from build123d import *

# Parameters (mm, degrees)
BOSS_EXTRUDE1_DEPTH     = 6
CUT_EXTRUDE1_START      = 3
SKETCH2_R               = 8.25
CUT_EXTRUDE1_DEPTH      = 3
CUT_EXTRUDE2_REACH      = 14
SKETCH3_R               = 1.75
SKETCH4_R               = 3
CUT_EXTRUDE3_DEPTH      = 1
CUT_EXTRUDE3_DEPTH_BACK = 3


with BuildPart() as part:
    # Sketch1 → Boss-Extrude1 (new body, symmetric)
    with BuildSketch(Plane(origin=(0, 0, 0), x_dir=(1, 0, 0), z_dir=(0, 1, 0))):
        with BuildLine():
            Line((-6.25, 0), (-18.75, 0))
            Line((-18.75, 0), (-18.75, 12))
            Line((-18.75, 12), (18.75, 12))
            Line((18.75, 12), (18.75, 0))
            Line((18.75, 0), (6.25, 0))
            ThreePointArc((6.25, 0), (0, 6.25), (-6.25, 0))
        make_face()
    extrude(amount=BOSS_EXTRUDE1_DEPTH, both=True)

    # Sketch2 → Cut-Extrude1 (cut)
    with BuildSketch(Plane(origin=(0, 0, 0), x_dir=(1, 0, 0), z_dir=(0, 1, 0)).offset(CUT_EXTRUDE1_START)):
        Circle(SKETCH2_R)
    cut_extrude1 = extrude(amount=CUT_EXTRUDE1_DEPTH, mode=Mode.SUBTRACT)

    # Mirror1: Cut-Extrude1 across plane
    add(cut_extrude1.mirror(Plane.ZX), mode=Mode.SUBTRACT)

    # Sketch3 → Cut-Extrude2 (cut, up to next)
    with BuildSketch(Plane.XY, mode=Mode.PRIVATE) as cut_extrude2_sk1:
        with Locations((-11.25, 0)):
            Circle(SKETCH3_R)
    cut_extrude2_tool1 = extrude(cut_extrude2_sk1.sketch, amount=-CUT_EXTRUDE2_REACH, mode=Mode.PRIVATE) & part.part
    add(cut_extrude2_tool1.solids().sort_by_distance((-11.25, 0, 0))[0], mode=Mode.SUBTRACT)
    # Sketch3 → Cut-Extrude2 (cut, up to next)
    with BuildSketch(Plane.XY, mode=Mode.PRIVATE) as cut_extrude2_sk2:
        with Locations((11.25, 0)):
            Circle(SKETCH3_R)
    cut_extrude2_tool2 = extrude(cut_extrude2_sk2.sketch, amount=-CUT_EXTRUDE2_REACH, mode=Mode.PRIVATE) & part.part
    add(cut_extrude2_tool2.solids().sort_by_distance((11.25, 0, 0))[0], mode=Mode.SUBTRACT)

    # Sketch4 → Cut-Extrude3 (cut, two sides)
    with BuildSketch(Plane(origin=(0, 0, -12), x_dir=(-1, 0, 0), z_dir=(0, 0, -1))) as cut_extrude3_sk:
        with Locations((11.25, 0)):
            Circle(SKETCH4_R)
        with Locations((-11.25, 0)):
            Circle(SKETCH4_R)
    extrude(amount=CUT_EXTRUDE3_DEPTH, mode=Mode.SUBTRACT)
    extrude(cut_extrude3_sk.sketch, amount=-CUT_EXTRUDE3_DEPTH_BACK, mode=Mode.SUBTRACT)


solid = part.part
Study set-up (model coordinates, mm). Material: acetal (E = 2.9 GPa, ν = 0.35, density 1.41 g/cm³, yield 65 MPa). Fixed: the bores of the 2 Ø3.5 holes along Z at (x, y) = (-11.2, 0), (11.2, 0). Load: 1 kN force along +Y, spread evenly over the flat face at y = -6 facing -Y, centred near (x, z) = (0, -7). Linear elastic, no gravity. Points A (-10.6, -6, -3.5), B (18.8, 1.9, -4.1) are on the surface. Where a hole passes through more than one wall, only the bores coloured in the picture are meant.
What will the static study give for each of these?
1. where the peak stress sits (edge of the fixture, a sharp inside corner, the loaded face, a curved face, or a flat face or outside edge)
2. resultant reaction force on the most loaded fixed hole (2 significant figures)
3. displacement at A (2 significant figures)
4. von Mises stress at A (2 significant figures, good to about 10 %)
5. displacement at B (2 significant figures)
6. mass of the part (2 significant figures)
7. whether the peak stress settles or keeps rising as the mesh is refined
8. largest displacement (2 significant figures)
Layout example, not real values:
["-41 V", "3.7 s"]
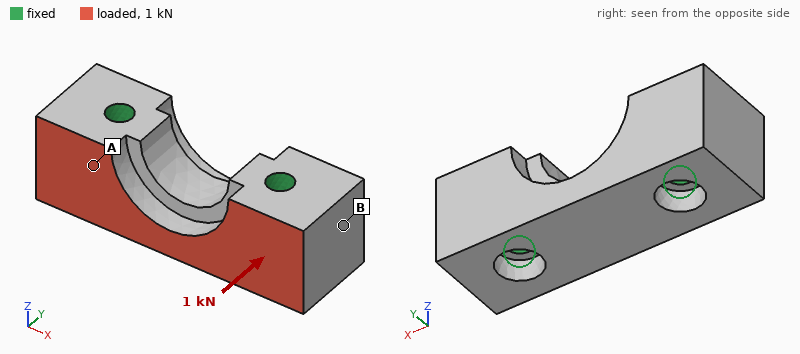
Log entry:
["edge of the fixture", "500 N", "8.7 µm", "5.6 MPa", "12 µm", "5.7 g", "keeps rising", "38 µm"]
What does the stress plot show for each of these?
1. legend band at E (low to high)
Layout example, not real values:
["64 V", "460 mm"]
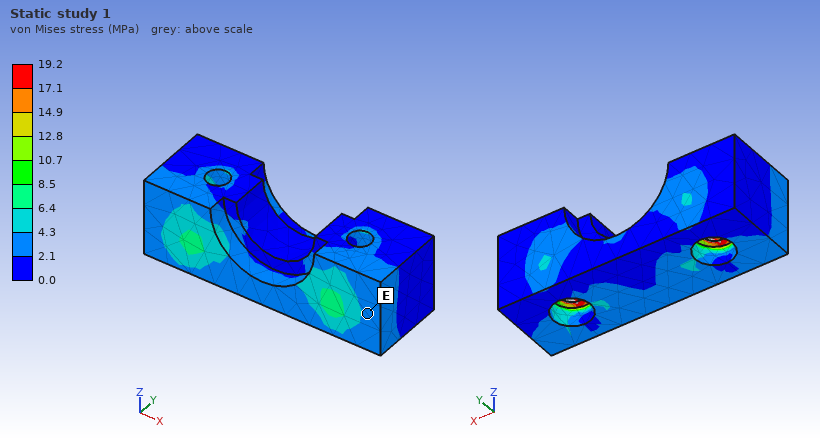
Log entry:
["2.1 to 4.3 MPa"]
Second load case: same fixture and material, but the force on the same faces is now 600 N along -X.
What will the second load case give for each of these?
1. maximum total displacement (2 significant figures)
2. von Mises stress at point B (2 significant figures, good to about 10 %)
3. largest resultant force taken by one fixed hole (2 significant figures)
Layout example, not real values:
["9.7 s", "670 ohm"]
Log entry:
["38 µm", "1.6 MPa", "310 N"]
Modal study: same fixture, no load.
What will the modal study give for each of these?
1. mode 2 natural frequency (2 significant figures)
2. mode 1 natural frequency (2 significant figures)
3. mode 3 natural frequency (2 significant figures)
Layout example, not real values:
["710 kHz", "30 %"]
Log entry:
["15 kHz", "12 kHz", "15 kHz"]
